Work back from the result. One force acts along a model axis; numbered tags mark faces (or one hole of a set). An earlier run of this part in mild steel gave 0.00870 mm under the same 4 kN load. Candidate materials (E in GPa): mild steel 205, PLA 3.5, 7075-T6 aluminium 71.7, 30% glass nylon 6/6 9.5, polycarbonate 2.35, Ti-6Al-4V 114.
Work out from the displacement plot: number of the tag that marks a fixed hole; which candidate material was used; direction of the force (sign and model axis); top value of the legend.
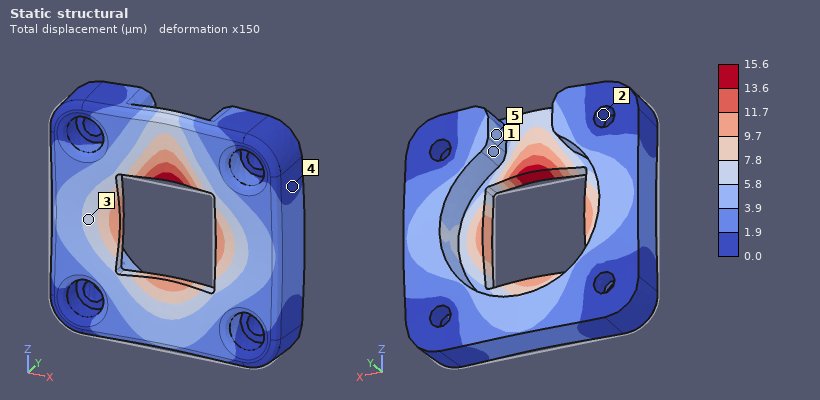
2
Ti-6Al-4V
+Y
15.6 µm
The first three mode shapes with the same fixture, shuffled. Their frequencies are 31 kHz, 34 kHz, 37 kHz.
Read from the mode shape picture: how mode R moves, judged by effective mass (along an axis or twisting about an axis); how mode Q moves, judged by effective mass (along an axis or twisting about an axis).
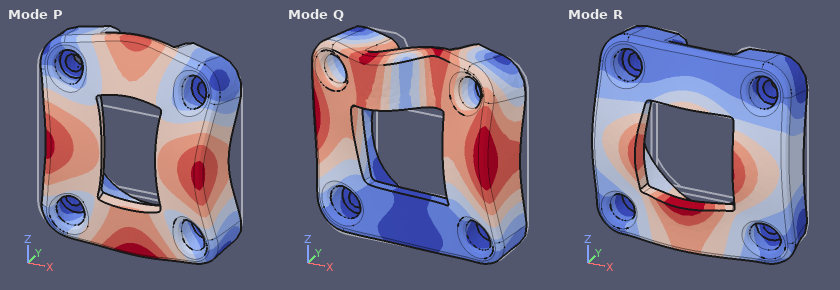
along Y
along X
